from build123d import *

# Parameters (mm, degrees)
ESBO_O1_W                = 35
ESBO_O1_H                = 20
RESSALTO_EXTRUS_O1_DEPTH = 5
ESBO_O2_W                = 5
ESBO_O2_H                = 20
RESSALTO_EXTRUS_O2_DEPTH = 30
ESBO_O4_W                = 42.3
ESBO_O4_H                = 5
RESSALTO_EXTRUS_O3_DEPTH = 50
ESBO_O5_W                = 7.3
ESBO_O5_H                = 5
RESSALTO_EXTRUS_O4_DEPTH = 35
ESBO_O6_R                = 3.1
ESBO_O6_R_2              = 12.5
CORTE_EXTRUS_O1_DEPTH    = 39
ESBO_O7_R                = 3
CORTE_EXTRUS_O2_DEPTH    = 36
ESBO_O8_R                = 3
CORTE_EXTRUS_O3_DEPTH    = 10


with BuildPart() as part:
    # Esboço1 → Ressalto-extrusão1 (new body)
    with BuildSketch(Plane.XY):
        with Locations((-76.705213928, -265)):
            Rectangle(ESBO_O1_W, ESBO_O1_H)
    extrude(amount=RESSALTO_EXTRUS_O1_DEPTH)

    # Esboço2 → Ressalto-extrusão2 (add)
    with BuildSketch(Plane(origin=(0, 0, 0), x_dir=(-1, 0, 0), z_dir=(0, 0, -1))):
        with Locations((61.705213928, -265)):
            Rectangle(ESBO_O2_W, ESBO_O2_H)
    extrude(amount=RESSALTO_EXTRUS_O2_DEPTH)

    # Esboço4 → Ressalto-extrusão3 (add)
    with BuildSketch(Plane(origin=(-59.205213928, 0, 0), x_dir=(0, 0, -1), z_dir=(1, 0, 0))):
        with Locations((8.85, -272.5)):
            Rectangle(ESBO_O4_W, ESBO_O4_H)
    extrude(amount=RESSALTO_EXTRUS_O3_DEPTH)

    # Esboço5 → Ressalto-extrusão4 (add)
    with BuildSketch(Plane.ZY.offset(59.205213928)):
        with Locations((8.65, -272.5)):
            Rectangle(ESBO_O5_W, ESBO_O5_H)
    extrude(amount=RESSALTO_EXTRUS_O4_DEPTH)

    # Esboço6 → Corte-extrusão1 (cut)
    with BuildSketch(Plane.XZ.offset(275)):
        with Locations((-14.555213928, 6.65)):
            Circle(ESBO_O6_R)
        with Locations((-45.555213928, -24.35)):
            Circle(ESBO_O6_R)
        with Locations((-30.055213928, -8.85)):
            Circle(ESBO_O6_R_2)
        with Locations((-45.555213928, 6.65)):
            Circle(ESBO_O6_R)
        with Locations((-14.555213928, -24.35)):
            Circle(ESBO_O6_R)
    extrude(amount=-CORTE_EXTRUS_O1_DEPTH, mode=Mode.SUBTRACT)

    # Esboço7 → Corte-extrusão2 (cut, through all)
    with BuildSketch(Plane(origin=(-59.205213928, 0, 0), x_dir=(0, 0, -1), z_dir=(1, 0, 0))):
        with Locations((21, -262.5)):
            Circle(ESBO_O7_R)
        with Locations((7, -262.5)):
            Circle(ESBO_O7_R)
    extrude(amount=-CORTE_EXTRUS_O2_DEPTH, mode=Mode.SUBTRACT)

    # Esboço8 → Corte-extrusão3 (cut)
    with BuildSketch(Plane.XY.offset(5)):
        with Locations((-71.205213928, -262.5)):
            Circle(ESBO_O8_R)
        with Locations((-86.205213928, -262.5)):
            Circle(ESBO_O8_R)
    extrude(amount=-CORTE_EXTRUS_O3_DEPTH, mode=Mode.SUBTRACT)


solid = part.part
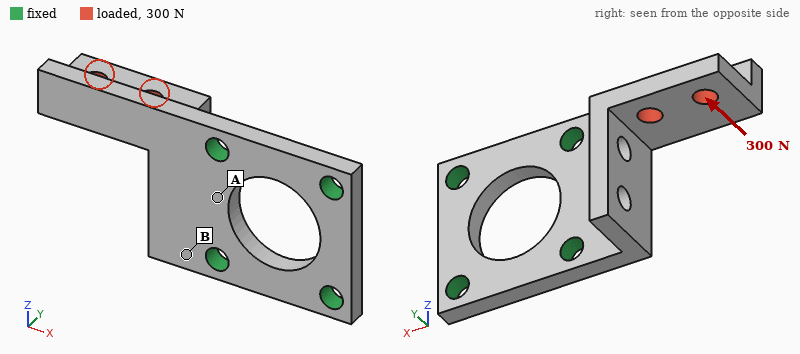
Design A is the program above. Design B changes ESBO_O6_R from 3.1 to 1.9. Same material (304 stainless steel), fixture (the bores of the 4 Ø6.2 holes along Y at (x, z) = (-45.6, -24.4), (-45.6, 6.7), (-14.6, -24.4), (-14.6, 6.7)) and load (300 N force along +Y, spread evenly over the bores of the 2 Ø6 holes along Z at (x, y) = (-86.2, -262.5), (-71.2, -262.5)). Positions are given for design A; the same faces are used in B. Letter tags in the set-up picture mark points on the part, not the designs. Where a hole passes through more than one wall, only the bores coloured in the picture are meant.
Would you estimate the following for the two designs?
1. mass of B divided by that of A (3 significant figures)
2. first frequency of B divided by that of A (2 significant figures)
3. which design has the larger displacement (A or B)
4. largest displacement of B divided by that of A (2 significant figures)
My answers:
1.03
0.92
B
1.2
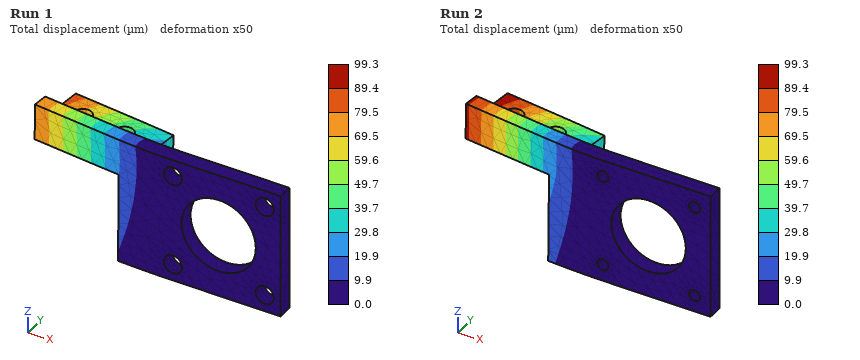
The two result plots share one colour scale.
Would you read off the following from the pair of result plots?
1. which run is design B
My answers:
Run 2
